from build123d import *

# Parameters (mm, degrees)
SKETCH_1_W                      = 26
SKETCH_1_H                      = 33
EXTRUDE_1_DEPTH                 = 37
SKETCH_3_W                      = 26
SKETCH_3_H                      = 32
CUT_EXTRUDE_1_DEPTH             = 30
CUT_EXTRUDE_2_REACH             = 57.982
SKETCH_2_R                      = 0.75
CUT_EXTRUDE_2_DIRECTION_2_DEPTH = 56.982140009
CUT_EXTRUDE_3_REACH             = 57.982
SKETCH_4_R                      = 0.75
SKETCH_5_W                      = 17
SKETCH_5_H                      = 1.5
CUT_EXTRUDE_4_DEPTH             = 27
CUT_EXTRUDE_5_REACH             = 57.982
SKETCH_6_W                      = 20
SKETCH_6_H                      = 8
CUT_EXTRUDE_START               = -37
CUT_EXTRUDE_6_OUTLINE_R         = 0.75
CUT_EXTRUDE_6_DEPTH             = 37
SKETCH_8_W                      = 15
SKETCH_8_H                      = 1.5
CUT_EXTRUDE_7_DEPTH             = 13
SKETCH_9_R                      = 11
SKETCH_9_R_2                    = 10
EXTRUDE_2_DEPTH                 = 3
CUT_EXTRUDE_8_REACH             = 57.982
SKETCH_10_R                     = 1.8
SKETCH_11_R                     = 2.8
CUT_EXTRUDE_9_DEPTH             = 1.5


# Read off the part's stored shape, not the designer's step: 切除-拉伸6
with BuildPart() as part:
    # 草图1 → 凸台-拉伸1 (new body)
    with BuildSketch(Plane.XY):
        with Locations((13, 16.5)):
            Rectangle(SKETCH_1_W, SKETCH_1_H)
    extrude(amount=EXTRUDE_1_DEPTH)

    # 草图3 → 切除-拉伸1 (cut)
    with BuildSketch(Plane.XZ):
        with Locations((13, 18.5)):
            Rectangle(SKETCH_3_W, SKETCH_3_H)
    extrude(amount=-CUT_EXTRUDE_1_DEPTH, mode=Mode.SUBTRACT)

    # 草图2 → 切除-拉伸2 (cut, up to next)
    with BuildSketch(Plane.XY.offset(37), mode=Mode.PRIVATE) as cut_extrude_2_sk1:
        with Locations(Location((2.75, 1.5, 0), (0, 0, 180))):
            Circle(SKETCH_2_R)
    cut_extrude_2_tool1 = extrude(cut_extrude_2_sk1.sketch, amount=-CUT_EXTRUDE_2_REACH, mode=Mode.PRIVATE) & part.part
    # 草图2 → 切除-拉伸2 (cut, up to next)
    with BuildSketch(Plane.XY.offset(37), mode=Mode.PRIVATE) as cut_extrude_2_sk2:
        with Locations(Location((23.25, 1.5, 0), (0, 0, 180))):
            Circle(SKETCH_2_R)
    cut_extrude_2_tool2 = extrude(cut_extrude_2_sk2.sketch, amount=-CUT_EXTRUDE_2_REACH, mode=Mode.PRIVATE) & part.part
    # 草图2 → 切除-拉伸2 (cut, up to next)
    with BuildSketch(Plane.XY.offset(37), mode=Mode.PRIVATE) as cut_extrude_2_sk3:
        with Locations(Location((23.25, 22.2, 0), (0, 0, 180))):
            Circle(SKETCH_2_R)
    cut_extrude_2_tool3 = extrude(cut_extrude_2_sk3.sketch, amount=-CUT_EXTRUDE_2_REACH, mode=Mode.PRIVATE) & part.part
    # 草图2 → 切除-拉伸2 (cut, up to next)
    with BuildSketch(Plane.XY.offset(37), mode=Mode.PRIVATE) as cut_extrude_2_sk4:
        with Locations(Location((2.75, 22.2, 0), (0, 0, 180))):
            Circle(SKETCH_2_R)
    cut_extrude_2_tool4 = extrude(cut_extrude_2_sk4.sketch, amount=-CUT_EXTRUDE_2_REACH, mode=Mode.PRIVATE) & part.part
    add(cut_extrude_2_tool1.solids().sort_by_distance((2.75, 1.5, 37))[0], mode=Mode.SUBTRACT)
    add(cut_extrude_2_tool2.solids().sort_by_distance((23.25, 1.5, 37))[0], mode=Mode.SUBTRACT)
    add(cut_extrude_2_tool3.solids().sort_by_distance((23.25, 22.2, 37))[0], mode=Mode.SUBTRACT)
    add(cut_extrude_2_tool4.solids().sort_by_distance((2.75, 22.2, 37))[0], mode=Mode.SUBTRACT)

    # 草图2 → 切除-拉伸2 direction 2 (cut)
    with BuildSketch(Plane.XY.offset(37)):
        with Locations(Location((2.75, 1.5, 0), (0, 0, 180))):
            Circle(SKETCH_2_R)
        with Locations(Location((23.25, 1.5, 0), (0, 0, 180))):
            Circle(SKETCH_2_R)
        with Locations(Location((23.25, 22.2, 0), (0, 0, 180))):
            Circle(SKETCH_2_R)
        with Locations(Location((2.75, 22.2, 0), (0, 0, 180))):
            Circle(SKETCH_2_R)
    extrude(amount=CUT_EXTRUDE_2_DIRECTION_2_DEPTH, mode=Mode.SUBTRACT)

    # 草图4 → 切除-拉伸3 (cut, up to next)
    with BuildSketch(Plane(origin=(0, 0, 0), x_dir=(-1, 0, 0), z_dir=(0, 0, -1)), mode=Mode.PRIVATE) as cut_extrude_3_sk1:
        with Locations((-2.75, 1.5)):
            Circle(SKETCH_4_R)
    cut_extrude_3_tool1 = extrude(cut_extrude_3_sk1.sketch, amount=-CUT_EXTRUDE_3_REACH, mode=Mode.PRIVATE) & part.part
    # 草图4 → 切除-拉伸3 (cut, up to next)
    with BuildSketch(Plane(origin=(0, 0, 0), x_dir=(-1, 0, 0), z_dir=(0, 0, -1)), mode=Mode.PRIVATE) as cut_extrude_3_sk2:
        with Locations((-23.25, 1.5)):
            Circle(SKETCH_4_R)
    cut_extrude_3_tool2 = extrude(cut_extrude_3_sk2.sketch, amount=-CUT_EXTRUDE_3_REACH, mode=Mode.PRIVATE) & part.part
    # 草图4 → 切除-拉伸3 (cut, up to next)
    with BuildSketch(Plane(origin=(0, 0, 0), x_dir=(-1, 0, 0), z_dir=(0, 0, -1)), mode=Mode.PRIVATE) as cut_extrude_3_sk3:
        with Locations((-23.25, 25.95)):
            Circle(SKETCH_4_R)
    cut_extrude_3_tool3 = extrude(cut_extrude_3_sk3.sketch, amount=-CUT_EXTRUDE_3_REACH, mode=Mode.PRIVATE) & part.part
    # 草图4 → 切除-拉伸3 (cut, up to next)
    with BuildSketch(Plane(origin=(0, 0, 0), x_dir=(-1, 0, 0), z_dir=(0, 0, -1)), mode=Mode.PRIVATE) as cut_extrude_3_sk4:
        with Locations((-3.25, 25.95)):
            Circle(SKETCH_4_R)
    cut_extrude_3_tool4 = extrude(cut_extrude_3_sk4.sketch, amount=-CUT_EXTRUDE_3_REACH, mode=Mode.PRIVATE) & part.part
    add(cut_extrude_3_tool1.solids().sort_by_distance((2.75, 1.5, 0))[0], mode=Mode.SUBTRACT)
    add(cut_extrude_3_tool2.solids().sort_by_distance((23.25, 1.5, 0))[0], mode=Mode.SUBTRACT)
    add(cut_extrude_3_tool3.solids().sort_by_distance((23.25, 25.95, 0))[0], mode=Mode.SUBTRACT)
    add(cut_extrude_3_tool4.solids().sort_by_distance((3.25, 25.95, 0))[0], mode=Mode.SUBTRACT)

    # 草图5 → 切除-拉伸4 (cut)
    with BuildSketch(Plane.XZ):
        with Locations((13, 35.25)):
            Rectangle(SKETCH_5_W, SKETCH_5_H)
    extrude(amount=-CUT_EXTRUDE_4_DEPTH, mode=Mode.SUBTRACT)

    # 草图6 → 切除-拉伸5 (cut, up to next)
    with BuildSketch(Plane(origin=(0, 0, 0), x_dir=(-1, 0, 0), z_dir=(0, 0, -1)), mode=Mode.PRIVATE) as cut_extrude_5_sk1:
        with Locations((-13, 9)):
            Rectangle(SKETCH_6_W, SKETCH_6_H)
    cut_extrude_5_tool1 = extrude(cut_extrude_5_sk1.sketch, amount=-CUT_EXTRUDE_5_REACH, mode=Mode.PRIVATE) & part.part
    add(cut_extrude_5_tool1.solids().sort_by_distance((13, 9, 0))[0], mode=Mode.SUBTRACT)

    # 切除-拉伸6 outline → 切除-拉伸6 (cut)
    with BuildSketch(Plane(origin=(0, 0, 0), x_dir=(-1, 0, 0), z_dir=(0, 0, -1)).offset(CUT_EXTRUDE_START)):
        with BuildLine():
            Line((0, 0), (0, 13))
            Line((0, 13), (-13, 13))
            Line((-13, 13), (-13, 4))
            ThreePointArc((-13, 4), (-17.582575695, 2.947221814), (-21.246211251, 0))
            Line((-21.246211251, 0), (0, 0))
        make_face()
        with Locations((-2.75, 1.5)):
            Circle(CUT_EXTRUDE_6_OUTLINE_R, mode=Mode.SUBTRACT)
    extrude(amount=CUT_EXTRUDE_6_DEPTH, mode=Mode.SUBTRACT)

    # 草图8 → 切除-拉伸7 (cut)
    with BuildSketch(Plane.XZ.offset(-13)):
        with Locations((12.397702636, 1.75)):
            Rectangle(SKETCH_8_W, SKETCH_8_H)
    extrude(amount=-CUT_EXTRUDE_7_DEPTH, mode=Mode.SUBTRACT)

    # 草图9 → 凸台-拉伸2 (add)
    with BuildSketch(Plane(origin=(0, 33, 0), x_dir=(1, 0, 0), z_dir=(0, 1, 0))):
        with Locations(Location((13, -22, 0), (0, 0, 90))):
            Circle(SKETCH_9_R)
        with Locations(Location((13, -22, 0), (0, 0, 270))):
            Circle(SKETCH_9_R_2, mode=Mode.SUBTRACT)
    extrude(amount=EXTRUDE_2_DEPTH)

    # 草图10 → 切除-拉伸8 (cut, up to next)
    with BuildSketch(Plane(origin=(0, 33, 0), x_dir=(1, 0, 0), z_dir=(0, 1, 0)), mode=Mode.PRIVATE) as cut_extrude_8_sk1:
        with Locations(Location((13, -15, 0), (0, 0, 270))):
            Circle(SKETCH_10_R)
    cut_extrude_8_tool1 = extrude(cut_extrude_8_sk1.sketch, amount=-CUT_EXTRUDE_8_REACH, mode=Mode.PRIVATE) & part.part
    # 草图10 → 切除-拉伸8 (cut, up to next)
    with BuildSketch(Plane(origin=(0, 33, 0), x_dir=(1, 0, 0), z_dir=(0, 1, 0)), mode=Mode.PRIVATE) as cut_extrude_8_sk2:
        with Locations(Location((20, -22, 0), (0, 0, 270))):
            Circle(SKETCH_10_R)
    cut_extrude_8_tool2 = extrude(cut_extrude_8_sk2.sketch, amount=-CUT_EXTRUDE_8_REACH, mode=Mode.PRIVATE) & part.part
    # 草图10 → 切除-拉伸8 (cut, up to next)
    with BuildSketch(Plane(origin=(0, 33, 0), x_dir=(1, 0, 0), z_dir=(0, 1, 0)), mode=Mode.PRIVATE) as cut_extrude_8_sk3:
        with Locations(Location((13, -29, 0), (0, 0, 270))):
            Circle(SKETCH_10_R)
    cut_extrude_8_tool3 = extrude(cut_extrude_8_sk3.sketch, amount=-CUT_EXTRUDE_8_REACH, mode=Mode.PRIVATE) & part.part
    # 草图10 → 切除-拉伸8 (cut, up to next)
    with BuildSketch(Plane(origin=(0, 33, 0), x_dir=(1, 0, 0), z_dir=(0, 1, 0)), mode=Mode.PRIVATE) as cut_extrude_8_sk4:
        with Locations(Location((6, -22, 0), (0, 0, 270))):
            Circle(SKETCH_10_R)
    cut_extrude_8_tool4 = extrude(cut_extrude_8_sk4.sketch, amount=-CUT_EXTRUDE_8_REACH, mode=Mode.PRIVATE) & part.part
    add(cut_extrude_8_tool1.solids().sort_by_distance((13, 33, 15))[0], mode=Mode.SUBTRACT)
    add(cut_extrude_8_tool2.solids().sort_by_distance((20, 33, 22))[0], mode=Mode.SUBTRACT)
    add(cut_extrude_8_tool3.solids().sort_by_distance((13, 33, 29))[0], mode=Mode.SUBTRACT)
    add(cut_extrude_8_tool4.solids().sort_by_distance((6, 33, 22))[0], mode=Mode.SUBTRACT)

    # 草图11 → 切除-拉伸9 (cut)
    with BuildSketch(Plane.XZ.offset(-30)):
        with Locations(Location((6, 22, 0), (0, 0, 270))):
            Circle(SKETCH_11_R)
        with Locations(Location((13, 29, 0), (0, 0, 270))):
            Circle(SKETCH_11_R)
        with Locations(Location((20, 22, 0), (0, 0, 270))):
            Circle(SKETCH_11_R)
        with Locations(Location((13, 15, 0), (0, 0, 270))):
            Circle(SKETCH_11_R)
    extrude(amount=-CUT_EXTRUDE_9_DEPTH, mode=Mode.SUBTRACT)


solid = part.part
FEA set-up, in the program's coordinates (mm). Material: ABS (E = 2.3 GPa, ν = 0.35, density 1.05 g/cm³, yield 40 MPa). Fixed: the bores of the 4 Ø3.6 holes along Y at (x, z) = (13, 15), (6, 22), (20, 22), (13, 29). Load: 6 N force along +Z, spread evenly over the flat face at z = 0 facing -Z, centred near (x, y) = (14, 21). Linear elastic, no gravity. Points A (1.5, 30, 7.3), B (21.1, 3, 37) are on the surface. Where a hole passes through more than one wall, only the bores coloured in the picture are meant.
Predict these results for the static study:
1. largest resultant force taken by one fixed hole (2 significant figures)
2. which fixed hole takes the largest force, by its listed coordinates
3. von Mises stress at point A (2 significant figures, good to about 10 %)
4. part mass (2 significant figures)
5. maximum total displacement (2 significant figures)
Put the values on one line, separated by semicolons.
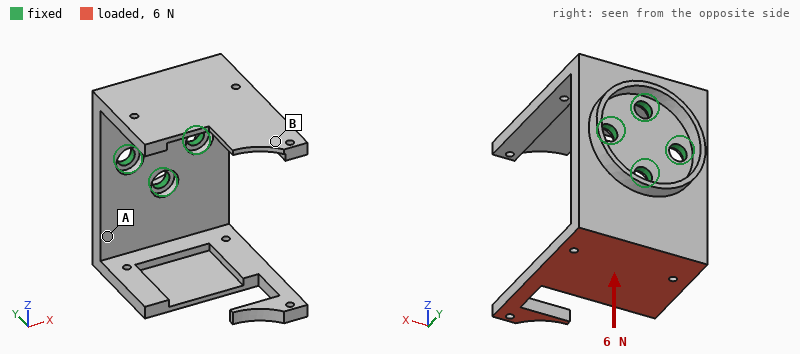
6.9 N; (13, 15); 1.5 MPa; 5.0 g; 0.57 mm
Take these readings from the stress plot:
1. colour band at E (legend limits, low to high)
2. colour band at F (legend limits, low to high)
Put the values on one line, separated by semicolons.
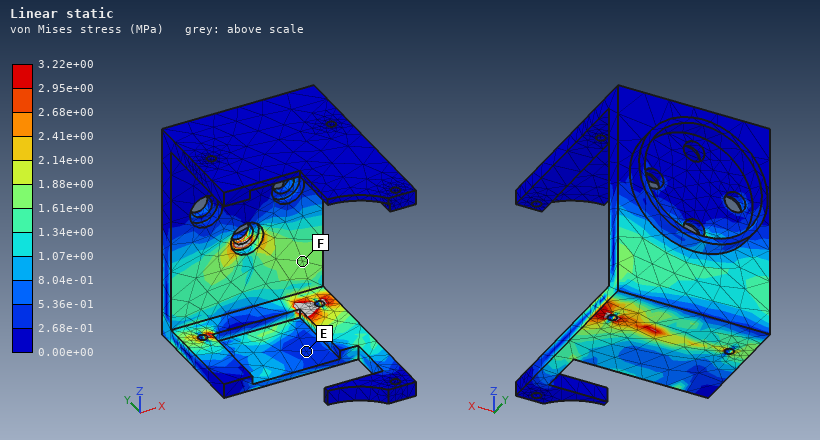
2.68e-01 to 5.36e-01 MPa; 1.61e+00 to 1.88e+00 MPa
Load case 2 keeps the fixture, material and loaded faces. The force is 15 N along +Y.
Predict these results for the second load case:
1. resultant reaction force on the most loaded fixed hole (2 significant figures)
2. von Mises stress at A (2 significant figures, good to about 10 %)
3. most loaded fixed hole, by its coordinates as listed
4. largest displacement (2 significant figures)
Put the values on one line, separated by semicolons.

35 N; 2.8 MPa; (13, 15); 0.61 mm
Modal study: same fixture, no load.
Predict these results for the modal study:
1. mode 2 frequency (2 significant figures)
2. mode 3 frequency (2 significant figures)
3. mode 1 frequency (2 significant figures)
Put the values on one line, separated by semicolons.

610 Hz; 990 Hz; 590 Hz
